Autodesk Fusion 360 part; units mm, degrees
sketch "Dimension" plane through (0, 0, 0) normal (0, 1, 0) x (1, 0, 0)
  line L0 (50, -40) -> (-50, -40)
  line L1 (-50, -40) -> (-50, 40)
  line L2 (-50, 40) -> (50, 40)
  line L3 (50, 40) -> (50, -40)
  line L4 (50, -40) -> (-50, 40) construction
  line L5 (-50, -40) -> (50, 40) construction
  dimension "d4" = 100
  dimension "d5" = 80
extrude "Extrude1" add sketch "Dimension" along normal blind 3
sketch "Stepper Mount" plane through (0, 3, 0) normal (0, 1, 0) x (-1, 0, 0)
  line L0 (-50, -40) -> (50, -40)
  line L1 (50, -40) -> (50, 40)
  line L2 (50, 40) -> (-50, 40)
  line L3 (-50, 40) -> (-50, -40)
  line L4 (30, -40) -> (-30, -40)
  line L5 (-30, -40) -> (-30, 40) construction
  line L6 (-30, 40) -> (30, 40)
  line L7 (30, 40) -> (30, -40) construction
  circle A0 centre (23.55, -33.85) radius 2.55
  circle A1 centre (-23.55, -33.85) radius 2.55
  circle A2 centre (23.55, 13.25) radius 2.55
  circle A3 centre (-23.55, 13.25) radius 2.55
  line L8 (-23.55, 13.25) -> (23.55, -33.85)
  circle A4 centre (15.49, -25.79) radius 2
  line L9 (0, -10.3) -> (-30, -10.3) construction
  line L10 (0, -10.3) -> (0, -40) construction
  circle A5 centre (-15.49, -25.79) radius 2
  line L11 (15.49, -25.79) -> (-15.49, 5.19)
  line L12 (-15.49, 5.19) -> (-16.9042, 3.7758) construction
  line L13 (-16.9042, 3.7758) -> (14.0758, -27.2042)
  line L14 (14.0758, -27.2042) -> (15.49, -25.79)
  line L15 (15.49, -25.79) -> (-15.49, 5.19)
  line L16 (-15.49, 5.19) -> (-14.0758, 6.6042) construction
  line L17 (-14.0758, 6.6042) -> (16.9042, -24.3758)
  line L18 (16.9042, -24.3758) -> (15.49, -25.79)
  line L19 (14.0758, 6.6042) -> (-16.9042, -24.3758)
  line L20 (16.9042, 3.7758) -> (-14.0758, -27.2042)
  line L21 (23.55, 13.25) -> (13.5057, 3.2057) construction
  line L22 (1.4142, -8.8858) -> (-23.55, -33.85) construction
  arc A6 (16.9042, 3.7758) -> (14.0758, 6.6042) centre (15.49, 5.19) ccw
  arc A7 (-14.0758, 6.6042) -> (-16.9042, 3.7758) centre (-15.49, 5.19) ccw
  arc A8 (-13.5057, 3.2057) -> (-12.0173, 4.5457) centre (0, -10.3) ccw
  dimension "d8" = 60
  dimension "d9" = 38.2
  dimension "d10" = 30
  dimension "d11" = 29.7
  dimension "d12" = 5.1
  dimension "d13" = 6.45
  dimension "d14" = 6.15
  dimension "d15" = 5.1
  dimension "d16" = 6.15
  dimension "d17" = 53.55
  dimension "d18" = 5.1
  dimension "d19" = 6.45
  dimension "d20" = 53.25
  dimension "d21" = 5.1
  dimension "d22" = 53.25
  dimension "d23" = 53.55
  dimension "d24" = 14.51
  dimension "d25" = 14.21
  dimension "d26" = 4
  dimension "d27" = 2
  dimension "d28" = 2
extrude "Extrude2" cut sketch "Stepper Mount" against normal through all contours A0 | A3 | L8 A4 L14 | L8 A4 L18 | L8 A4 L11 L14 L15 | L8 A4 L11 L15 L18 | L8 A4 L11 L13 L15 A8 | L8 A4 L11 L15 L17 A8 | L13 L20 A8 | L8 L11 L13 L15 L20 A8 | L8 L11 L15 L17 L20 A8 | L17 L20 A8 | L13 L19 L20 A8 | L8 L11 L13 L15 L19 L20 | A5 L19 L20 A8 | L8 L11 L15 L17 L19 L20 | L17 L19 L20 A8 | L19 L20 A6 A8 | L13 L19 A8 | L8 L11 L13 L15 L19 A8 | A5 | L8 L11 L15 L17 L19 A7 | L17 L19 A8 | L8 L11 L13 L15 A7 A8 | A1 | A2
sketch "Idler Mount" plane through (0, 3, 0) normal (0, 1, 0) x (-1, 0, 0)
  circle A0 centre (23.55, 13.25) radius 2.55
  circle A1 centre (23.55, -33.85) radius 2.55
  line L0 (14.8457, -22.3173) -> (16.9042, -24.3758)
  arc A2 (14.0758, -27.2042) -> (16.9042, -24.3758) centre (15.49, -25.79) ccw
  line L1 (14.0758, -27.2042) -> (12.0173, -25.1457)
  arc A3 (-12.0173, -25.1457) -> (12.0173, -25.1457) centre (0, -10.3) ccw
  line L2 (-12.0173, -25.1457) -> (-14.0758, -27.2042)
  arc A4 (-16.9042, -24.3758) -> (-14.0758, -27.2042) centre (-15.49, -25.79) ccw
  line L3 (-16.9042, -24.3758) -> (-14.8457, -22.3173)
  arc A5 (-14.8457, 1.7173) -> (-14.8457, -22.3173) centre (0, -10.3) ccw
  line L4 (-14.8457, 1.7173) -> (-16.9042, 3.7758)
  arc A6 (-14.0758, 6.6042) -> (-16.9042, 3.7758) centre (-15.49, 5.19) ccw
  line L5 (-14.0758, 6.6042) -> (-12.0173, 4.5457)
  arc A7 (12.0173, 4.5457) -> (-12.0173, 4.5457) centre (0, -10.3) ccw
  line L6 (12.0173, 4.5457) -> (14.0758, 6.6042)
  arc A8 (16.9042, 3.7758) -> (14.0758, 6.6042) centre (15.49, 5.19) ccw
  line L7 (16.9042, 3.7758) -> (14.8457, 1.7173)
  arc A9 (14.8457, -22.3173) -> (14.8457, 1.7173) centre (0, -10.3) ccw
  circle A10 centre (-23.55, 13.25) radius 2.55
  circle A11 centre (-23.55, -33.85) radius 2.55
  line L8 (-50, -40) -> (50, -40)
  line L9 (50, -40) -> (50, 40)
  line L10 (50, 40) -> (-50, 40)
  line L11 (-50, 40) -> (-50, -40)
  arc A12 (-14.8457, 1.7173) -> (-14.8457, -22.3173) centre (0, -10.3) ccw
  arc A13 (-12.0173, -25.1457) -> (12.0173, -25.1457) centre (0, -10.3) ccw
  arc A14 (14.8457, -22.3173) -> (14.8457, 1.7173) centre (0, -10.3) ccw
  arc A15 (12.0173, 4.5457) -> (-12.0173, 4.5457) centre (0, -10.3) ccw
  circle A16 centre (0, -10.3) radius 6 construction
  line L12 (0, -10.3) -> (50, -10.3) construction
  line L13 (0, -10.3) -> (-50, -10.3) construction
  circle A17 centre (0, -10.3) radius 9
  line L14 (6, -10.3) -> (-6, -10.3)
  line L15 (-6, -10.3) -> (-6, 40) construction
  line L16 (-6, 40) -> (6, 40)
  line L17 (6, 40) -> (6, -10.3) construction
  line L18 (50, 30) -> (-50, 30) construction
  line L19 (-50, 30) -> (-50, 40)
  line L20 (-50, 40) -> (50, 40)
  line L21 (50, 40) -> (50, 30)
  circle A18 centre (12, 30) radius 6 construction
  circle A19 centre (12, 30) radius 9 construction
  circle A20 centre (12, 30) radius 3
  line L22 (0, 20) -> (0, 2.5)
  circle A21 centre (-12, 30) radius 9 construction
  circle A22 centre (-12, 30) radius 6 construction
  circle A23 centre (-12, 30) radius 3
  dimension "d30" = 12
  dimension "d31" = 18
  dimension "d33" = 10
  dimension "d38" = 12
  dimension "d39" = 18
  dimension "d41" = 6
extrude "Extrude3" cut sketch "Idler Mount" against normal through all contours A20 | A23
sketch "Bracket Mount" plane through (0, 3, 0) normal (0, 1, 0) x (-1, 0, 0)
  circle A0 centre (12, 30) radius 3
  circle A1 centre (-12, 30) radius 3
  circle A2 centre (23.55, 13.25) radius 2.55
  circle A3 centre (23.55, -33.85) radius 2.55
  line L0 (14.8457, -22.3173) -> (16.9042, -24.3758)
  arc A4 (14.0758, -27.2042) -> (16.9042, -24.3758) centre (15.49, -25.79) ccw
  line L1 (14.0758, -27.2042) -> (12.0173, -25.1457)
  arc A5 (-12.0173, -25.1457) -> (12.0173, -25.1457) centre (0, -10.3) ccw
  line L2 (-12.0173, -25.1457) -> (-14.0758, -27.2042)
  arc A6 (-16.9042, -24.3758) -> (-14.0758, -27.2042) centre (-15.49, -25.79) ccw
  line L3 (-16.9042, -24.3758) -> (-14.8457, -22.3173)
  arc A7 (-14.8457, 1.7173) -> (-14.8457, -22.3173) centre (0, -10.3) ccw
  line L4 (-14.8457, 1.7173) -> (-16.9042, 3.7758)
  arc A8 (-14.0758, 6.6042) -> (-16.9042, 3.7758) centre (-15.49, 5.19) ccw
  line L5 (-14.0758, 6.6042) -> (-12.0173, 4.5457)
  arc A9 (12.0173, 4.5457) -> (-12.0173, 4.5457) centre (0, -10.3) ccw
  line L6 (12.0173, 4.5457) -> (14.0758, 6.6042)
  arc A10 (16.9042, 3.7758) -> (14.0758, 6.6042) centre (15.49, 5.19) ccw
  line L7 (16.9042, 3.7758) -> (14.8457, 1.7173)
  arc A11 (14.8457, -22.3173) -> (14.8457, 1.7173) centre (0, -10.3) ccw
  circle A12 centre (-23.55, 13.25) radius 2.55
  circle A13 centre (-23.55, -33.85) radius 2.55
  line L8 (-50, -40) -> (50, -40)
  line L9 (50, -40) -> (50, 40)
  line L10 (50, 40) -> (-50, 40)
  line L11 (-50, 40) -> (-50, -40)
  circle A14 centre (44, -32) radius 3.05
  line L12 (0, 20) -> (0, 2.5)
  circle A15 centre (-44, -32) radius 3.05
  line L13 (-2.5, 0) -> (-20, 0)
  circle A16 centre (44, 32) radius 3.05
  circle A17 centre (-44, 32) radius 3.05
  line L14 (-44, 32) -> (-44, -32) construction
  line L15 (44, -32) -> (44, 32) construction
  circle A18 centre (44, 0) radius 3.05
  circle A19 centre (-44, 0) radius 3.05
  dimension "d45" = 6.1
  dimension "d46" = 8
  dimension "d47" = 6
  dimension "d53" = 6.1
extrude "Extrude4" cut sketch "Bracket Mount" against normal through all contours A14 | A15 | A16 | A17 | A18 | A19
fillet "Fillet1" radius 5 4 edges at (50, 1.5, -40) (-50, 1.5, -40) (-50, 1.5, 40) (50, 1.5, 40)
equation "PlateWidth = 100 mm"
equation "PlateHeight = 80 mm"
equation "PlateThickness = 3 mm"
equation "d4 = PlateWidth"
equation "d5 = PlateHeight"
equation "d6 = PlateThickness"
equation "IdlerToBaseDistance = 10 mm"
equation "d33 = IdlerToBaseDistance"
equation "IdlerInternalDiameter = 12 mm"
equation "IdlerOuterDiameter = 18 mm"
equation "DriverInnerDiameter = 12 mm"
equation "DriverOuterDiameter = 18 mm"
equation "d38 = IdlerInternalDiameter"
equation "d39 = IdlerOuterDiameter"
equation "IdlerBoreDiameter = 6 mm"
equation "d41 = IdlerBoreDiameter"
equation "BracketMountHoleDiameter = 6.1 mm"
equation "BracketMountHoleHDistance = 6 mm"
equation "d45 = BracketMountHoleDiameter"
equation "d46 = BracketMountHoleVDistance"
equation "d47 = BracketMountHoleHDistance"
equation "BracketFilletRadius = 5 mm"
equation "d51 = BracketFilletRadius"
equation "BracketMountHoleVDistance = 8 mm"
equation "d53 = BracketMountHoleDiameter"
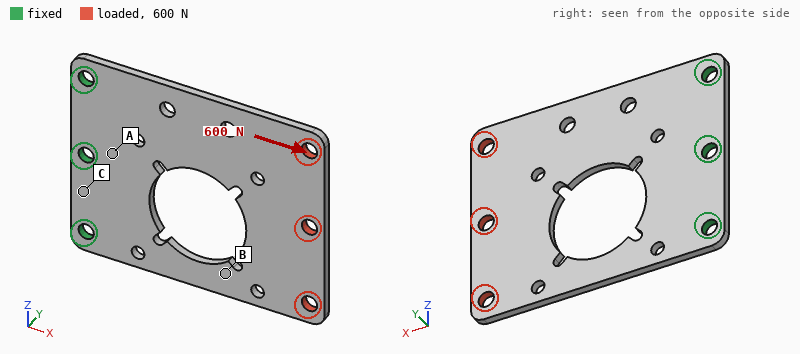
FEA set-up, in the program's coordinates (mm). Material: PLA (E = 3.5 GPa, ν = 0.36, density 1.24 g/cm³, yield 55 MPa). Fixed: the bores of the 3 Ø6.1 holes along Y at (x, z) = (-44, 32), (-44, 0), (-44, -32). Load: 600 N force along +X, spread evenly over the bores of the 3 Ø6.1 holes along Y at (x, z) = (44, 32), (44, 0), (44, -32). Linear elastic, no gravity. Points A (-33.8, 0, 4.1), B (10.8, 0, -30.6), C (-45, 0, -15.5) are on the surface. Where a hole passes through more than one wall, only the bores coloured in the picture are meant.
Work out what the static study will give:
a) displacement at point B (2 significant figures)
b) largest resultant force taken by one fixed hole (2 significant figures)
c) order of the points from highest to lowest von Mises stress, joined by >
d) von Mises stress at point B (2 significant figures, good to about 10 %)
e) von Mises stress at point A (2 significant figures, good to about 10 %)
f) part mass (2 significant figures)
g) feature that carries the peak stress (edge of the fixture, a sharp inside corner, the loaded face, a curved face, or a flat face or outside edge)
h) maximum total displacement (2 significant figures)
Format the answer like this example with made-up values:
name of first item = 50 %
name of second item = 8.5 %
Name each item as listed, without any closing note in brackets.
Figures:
displacement at point B = 0.12 mm
largest resultant force taken by one fixed hole = 230 N
order of the points from highest to lowest von Mises stress, joined by > = B > A > C
von Mises stress at point B = 7.2 MPa
von Mises stress at point A = 3.3 MPa
part mass = 24 g
feature that carries the peak stress = a curved face
maximum total displacement = 0.18 mm
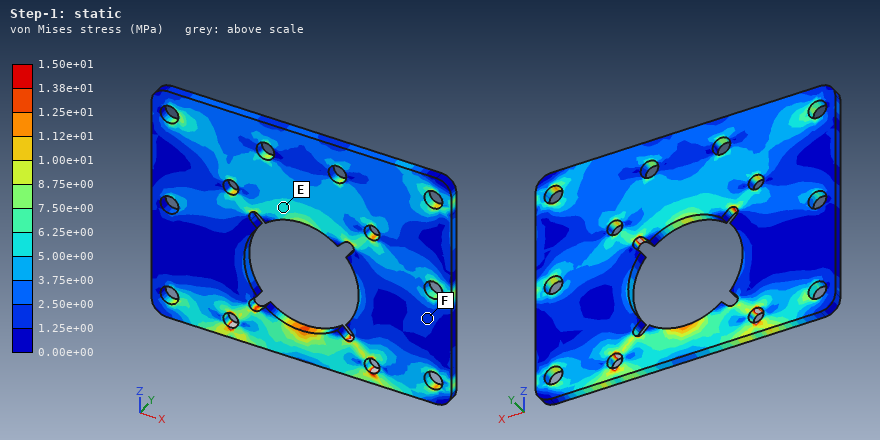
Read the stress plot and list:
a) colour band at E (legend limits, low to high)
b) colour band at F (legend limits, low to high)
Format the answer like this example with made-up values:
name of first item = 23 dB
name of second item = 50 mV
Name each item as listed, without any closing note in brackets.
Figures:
colour band at E = 5.00e+00 to 6.25e+00 MPa
colour band at F = 1.25e+00 to 2.50e+00 MPa
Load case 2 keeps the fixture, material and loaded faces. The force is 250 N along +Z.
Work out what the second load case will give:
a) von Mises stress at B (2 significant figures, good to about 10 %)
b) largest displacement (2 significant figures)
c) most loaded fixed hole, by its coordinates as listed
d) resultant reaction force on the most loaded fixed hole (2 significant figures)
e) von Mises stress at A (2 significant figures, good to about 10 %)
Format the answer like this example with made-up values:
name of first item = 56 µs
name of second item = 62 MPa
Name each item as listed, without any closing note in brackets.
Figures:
von Mises stress at B = 8.5 MPa
largest displacement = 0.53 mm
most loaded fixed hole, by its coordinates as listed = (-44, 32)
resultant reaction force on the most loaded fixed hole = 380 N
von Mises stress at A = 4.8 MPa
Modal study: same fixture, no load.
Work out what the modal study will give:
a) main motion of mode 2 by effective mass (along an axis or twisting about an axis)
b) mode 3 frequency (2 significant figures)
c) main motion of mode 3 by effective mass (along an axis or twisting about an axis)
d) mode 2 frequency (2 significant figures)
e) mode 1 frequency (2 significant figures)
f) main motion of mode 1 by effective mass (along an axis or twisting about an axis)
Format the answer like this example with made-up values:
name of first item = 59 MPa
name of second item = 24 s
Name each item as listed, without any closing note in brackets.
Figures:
main motion of mode 2 by effective mass = twisting about X
mode 3 frequency = 570 Hz
main motion of mode 3 by effective mass = along Y
mode 2 frequency = 230 Hz
mode 1 frequency = 85 Hz
main motion of mode 1 by effective mass = along Y
